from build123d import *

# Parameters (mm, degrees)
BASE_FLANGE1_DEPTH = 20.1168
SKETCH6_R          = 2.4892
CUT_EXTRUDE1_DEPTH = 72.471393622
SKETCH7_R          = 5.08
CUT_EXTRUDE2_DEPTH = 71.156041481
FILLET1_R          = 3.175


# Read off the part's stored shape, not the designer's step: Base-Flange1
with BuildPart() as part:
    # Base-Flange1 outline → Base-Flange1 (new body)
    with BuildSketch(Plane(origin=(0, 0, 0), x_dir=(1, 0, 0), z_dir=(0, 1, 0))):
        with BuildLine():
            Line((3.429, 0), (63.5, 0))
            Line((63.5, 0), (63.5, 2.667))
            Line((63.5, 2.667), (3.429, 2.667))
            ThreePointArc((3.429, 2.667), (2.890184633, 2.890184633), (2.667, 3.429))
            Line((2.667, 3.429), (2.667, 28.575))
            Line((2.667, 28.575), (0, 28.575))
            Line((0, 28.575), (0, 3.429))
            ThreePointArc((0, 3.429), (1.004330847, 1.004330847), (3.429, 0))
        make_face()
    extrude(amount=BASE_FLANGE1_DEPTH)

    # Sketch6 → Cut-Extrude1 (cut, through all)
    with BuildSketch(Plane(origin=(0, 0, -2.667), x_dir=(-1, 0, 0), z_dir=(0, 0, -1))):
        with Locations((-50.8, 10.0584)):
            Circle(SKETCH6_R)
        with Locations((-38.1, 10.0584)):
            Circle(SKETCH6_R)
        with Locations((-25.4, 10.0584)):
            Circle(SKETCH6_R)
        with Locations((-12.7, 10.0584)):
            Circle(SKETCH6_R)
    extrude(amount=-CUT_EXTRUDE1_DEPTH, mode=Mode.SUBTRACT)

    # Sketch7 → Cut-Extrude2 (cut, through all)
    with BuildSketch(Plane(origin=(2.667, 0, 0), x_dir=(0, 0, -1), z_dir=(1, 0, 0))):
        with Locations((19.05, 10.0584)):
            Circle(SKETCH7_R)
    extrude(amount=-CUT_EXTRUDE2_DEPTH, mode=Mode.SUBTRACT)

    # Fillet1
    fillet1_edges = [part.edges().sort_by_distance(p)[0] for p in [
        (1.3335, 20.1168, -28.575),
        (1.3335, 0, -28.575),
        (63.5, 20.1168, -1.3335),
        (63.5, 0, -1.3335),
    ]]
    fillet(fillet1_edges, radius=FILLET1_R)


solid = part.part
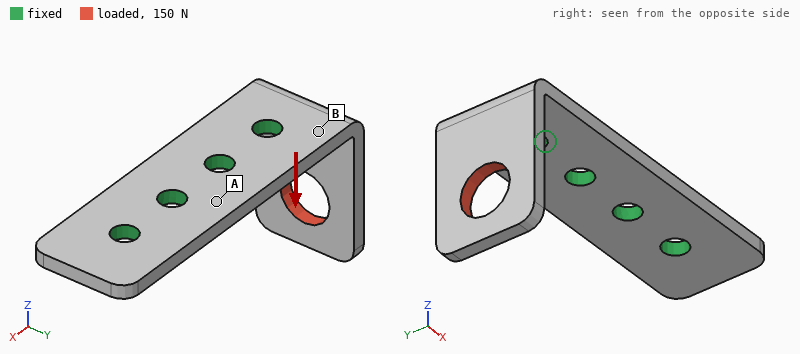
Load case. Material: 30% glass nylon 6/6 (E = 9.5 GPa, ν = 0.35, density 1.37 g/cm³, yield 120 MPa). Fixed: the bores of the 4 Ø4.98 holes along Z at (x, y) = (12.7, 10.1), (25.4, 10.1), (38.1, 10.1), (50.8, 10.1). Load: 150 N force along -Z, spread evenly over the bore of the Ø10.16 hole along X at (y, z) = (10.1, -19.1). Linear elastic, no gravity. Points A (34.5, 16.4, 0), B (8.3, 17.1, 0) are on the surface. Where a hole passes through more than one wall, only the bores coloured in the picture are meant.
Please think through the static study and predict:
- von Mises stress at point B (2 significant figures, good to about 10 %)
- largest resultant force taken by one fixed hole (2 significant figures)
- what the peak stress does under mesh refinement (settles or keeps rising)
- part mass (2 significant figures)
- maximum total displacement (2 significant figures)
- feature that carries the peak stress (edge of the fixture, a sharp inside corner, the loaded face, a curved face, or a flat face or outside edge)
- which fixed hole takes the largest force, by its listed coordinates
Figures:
31 MPa
170 N
keeps rising
5.9 g
0.74 mm
edge of the fixture
(12.7, 10.1)
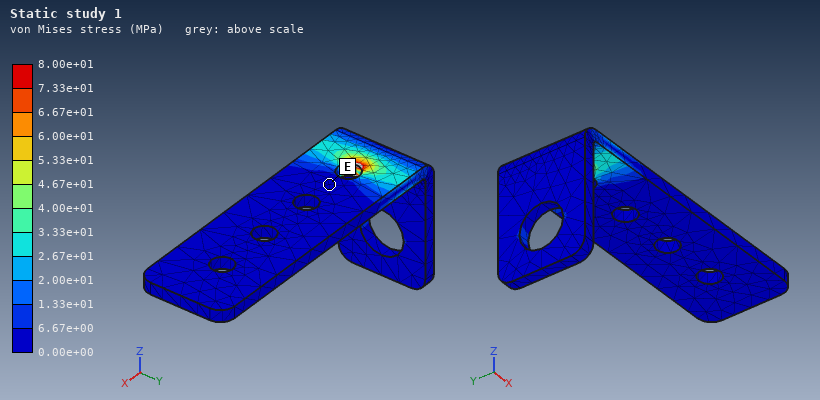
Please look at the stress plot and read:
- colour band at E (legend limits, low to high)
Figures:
0.00e+00 to 6.67e+00 MPa
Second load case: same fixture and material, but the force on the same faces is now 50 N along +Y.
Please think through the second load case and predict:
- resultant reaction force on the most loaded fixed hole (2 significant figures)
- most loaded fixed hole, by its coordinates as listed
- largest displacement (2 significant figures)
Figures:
69 N
(12.7, 10.1)
0.46 mm
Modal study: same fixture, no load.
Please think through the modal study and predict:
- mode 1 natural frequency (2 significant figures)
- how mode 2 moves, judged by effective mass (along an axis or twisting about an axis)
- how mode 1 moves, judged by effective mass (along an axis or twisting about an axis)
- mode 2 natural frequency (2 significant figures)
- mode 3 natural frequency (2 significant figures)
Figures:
1100 Hz
along Y
along X
1700 Hz
4000 Hz
